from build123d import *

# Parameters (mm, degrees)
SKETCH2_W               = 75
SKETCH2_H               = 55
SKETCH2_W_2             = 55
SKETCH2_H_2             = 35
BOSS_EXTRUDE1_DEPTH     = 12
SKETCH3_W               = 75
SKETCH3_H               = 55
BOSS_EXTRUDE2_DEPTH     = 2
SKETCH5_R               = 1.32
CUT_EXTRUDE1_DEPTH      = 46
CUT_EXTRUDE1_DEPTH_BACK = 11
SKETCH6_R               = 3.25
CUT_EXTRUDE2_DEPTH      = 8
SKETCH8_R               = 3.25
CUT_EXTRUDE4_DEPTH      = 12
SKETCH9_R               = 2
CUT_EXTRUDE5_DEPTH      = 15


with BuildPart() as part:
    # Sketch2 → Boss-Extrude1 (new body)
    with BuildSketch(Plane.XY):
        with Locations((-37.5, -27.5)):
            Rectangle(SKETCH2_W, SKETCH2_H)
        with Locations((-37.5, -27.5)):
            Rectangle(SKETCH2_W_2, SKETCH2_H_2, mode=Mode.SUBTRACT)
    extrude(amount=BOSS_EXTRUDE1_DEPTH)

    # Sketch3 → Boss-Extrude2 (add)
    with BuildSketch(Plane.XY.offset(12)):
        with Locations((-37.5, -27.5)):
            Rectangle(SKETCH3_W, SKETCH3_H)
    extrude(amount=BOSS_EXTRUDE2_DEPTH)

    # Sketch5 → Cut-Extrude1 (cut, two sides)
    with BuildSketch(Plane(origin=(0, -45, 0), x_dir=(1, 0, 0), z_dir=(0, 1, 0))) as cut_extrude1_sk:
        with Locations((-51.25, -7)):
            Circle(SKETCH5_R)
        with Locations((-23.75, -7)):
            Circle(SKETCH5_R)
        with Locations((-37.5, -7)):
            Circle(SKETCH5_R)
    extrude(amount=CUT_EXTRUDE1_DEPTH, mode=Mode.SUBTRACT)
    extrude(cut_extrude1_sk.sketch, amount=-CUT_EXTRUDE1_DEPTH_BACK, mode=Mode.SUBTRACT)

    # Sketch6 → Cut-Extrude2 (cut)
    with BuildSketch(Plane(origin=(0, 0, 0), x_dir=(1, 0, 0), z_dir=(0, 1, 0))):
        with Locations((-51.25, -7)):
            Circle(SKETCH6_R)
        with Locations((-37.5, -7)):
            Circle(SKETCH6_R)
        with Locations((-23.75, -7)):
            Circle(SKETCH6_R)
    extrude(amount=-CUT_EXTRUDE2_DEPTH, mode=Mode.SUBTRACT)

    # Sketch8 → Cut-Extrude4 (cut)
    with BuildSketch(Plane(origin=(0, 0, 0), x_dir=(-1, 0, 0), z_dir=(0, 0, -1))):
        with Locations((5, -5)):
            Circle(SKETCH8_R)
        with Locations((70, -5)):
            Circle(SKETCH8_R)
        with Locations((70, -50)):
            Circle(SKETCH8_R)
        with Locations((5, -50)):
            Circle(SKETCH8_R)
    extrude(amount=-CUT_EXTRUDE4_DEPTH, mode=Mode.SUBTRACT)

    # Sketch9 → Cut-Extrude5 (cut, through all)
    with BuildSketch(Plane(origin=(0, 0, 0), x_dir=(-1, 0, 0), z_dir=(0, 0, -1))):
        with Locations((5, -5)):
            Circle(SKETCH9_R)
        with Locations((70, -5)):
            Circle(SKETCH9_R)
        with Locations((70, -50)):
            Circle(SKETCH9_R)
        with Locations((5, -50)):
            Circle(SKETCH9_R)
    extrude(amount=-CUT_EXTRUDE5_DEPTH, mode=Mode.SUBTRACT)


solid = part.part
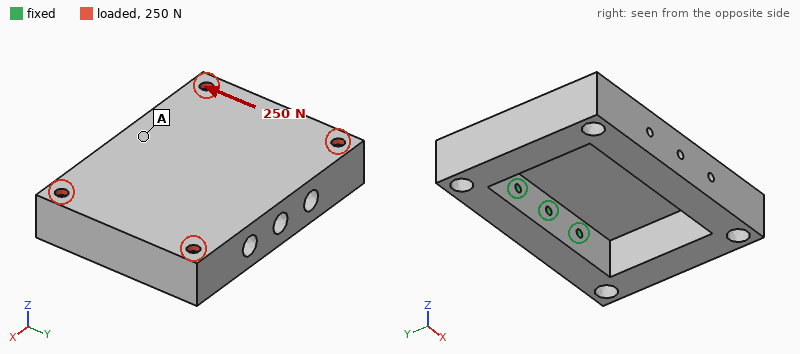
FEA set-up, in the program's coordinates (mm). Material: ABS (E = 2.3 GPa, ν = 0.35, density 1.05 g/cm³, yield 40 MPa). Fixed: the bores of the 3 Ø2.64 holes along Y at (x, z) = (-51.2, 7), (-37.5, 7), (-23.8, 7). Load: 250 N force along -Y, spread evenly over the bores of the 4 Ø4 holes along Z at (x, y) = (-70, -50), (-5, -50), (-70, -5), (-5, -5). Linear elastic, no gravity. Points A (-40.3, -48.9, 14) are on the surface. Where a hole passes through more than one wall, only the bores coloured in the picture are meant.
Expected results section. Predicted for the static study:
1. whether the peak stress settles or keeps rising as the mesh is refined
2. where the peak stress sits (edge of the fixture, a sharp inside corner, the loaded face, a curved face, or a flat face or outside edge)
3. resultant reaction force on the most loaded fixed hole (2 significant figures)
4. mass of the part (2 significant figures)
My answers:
keeps rising
edge of the fixture
96 N
34 g
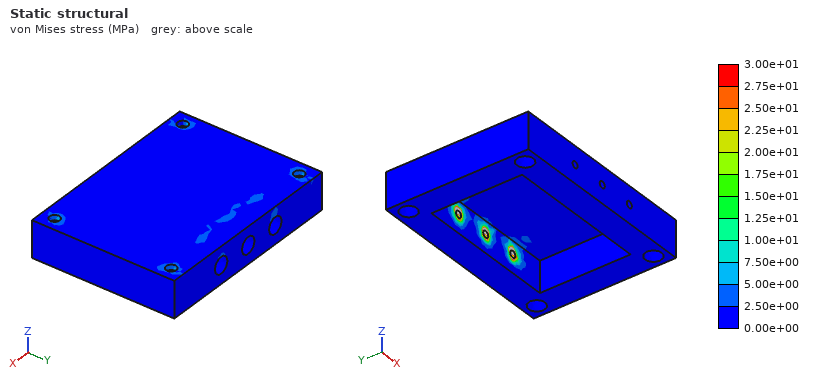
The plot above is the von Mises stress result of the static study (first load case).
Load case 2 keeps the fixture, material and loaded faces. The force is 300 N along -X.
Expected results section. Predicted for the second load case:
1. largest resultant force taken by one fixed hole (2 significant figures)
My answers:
240 N
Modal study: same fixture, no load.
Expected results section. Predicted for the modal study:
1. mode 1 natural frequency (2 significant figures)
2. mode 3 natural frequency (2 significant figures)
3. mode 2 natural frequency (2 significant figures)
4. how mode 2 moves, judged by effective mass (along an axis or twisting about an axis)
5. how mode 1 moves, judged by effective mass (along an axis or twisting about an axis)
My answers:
240 Hz
900 Hz
670 Hz
along X
along Z
